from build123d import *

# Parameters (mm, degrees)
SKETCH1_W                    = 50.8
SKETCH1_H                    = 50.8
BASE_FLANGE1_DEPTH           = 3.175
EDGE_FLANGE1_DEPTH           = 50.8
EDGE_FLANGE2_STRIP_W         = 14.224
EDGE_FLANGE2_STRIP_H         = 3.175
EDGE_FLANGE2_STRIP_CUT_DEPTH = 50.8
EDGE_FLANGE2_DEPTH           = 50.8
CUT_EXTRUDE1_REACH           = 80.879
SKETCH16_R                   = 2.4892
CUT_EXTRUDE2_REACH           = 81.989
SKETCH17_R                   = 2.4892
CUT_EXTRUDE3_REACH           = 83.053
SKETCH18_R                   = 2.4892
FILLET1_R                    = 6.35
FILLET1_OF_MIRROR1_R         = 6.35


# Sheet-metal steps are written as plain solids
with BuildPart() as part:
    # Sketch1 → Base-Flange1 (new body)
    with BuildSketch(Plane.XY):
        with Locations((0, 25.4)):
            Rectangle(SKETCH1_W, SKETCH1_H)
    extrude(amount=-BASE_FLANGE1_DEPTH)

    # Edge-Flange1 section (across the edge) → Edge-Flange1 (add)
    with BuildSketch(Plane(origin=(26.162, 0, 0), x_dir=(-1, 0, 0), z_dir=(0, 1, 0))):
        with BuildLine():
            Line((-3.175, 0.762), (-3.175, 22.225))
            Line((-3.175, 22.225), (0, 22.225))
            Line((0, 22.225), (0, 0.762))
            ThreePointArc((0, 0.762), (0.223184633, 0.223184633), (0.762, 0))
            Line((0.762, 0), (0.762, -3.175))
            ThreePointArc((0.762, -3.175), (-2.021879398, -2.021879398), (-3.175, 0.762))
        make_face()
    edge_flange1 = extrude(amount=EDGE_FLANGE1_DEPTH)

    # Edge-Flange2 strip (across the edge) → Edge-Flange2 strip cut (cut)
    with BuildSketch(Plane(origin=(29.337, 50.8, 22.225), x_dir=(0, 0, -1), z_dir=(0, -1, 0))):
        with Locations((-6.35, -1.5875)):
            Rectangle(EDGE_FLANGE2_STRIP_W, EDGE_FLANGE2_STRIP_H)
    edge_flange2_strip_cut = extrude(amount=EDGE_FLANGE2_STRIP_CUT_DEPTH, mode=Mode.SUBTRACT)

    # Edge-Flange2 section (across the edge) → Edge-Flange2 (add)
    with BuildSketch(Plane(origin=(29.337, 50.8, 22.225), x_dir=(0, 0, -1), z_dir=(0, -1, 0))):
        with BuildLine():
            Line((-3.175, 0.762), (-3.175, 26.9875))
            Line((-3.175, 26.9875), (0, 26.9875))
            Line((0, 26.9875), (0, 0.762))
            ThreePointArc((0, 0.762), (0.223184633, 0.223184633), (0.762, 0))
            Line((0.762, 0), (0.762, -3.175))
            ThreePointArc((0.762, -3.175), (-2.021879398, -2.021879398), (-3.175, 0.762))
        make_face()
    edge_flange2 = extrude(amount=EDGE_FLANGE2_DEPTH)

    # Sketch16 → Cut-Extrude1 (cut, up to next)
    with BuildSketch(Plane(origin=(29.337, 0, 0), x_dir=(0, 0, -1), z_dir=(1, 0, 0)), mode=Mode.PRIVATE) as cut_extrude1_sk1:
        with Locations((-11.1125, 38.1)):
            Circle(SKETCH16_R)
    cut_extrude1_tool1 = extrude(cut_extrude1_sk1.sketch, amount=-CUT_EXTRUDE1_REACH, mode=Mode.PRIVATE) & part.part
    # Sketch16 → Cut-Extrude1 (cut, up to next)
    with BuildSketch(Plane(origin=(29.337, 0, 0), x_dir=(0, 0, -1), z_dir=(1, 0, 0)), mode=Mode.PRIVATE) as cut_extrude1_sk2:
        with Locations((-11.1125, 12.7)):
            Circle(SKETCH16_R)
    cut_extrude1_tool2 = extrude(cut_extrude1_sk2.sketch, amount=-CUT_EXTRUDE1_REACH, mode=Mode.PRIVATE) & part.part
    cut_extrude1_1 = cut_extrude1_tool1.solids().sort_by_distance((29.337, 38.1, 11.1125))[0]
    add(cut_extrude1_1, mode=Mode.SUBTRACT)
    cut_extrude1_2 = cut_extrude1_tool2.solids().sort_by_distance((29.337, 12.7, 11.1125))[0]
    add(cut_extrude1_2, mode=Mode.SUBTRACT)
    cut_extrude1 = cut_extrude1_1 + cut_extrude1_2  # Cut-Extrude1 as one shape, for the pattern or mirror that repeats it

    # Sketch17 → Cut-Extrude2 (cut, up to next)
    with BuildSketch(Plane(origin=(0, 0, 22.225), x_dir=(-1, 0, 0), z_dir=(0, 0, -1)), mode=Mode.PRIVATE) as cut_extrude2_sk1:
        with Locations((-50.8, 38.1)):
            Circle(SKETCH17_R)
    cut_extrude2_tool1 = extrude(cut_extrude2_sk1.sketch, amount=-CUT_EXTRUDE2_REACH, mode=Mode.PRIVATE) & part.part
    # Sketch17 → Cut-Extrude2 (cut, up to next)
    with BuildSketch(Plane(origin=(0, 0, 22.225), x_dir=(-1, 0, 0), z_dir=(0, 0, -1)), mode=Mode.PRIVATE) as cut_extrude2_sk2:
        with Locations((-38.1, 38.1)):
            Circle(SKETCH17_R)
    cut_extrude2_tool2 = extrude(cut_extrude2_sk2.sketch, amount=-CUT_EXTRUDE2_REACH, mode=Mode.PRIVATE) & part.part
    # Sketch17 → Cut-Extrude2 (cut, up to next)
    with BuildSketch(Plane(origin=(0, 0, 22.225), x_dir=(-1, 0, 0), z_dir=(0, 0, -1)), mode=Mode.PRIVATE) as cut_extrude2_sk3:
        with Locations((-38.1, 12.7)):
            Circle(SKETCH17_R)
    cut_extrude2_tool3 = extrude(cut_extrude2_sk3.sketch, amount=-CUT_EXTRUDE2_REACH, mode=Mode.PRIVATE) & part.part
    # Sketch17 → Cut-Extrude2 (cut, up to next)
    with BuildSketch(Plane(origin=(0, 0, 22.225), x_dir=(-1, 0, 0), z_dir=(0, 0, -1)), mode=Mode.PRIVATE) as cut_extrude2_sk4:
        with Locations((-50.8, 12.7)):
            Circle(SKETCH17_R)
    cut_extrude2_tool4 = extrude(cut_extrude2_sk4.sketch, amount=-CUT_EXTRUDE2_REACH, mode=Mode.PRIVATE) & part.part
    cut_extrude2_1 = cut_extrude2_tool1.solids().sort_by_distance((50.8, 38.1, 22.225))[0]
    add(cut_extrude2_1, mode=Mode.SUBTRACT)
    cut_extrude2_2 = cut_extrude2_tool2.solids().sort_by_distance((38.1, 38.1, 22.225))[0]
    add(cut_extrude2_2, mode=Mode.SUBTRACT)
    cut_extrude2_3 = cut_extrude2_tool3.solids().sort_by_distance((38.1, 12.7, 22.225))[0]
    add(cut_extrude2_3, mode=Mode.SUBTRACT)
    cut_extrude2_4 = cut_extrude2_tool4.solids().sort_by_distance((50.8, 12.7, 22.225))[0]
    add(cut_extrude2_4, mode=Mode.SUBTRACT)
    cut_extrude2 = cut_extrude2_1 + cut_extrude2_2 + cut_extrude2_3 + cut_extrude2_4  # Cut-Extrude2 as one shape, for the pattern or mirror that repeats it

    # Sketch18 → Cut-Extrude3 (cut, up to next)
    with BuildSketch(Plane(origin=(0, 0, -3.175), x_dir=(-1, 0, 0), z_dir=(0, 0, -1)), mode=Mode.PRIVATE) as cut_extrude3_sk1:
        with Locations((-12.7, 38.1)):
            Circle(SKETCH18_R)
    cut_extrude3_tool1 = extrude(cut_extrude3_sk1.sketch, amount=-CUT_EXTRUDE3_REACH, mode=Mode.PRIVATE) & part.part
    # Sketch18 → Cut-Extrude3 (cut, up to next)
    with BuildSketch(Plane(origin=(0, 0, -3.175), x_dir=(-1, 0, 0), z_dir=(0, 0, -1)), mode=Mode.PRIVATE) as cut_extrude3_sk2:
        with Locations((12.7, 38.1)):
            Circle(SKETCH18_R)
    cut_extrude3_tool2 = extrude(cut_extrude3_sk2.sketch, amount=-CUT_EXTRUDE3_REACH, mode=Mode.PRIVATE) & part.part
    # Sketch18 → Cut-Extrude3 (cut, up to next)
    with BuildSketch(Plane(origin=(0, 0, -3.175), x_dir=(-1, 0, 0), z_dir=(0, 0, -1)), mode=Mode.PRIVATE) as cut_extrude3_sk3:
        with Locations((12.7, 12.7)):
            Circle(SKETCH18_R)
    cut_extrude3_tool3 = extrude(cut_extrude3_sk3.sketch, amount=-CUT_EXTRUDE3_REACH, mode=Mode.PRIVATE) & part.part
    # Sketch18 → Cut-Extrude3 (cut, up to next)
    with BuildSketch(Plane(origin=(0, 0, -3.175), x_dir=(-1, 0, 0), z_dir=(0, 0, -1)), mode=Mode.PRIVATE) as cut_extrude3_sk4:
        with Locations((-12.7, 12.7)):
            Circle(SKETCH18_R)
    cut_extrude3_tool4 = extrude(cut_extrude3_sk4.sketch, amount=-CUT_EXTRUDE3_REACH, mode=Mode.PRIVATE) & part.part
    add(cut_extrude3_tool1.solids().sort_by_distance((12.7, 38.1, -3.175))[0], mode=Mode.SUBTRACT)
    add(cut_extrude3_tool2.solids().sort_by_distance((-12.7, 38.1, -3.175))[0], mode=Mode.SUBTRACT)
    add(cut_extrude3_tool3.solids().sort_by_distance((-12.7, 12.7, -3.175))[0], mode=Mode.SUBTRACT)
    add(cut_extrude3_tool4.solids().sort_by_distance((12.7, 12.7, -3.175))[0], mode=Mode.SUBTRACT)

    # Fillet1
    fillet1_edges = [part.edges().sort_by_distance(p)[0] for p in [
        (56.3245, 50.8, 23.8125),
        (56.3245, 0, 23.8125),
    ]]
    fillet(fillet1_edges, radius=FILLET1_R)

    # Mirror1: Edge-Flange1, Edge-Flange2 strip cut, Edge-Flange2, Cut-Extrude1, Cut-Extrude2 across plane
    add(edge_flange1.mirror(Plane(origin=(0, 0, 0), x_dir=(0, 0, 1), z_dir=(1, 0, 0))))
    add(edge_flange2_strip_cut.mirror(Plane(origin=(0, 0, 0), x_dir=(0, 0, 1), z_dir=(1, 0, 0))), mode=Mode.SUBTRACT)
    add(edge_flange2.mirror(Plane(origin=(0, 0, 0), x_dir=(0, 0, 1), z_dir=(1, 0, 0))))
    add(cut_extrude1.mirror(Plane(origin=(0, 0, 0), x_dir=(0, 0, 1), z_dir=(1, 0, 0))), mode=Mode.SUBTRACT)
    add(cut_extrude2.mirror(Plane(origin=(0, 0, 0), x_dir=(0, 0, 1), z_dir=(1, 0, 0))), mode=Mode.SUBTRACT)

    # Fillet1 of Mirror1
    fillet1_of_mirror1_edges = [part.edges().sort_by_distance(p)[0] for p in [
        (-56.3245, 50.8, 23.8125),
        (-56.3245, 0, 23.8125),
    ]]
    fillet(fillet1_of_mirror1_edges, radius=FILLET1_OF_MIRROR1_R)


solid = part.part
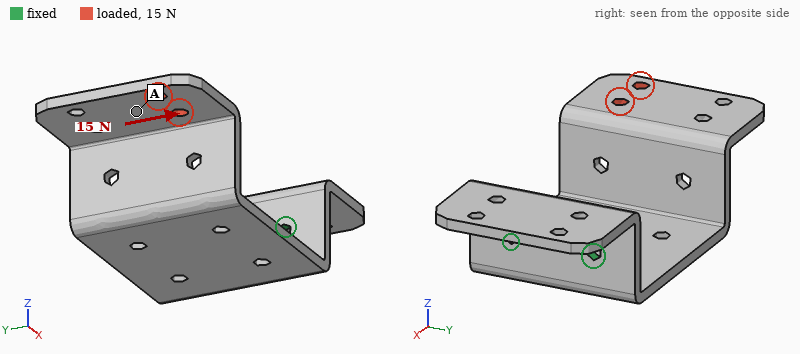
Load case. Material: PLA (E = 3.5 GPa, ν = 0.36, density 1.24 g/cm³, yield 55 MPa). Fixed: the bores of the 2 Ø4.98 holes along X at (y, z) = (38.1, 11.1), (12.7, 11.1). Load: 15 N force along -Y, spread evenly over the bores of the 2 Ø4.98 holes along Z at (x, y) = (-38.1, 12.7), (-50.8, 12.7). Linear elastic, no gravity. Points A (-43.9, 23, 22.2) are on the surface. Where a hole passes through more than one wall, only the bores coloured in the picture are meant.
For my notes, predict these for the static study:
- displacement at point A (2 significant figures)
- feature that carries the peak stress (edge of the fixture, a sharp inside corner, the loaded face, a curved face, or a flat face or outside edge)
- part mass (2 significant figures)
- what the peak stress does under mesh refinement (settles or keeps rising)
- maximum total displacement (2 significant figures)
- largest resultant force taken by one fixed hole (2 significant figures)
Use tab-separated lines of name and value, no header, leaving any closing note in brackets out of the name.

displacement at point A	1.1 mm
feature that carries the peak stress	edge of the fixture
part mass	31 g
what the peak stress does under mesh refinement	keeps rising
maximum total displacement	1.4 mm
largest resultant force taken by one fixed hole	37 N
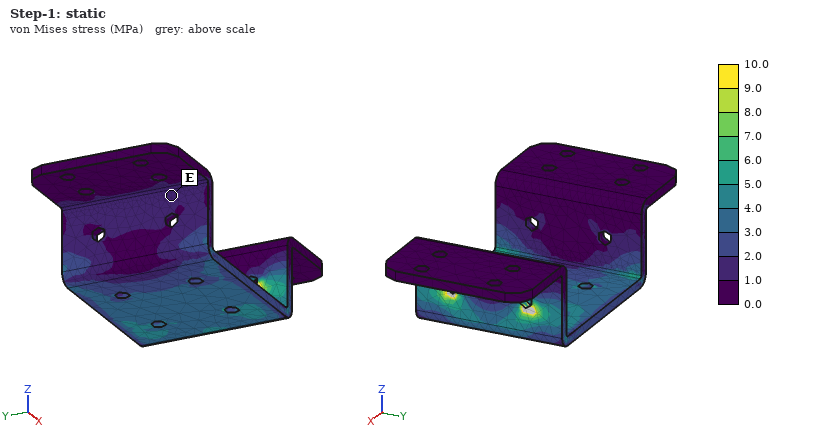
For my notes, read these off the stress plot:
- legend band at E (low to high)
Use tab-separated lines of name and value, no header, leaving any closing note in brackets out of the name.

legend band at E	1.0 to 2.0 MPa
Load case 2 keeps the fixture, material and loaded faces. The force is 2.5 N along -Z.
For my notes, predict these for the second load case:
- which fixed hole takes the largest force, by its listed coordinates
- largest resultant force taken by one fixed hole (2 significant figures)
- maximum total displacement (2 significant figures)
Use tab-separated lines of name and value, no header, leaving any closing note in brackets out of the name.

which fixed hole takes the largest force, by its listed coordinates	(12.7, 11.1)
largest resultant force taken by one fixed hole	2.5 N
maximum total displacement	1.3 mm
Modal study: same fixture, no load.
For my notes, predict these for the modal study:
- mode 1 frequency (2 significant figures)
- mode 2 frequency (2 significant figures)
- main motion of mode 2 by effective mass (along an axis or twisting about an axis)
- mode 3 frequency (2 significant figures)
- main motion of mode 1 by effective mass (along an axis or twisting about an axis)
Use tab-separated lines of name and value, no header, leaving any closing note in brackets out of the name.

mode 1 frequency	83 Hz
mode 2 frequency	190 Hz
main motion of mode 2 by effective mass	along Y
mode 3 frequency	340 Hz
main motion of mode 1 by effective mass	along Z
